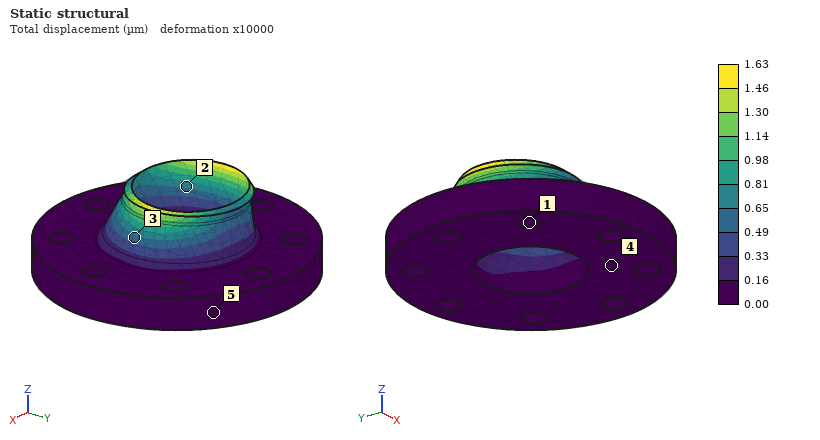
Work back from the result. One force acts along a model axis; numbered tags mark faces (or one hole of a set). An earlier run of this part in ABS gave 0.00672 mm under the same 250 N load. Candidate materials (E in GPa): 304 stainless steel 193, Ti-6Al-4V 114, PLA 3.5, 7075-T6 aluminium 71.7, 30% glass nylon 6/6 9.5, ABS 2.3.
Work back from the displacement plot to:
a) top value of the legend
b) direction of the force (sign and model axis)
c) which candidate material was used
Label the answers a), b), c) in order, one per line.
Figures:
a) 1.63 µm
b) -X
c) 30% glass nylon 6/6
